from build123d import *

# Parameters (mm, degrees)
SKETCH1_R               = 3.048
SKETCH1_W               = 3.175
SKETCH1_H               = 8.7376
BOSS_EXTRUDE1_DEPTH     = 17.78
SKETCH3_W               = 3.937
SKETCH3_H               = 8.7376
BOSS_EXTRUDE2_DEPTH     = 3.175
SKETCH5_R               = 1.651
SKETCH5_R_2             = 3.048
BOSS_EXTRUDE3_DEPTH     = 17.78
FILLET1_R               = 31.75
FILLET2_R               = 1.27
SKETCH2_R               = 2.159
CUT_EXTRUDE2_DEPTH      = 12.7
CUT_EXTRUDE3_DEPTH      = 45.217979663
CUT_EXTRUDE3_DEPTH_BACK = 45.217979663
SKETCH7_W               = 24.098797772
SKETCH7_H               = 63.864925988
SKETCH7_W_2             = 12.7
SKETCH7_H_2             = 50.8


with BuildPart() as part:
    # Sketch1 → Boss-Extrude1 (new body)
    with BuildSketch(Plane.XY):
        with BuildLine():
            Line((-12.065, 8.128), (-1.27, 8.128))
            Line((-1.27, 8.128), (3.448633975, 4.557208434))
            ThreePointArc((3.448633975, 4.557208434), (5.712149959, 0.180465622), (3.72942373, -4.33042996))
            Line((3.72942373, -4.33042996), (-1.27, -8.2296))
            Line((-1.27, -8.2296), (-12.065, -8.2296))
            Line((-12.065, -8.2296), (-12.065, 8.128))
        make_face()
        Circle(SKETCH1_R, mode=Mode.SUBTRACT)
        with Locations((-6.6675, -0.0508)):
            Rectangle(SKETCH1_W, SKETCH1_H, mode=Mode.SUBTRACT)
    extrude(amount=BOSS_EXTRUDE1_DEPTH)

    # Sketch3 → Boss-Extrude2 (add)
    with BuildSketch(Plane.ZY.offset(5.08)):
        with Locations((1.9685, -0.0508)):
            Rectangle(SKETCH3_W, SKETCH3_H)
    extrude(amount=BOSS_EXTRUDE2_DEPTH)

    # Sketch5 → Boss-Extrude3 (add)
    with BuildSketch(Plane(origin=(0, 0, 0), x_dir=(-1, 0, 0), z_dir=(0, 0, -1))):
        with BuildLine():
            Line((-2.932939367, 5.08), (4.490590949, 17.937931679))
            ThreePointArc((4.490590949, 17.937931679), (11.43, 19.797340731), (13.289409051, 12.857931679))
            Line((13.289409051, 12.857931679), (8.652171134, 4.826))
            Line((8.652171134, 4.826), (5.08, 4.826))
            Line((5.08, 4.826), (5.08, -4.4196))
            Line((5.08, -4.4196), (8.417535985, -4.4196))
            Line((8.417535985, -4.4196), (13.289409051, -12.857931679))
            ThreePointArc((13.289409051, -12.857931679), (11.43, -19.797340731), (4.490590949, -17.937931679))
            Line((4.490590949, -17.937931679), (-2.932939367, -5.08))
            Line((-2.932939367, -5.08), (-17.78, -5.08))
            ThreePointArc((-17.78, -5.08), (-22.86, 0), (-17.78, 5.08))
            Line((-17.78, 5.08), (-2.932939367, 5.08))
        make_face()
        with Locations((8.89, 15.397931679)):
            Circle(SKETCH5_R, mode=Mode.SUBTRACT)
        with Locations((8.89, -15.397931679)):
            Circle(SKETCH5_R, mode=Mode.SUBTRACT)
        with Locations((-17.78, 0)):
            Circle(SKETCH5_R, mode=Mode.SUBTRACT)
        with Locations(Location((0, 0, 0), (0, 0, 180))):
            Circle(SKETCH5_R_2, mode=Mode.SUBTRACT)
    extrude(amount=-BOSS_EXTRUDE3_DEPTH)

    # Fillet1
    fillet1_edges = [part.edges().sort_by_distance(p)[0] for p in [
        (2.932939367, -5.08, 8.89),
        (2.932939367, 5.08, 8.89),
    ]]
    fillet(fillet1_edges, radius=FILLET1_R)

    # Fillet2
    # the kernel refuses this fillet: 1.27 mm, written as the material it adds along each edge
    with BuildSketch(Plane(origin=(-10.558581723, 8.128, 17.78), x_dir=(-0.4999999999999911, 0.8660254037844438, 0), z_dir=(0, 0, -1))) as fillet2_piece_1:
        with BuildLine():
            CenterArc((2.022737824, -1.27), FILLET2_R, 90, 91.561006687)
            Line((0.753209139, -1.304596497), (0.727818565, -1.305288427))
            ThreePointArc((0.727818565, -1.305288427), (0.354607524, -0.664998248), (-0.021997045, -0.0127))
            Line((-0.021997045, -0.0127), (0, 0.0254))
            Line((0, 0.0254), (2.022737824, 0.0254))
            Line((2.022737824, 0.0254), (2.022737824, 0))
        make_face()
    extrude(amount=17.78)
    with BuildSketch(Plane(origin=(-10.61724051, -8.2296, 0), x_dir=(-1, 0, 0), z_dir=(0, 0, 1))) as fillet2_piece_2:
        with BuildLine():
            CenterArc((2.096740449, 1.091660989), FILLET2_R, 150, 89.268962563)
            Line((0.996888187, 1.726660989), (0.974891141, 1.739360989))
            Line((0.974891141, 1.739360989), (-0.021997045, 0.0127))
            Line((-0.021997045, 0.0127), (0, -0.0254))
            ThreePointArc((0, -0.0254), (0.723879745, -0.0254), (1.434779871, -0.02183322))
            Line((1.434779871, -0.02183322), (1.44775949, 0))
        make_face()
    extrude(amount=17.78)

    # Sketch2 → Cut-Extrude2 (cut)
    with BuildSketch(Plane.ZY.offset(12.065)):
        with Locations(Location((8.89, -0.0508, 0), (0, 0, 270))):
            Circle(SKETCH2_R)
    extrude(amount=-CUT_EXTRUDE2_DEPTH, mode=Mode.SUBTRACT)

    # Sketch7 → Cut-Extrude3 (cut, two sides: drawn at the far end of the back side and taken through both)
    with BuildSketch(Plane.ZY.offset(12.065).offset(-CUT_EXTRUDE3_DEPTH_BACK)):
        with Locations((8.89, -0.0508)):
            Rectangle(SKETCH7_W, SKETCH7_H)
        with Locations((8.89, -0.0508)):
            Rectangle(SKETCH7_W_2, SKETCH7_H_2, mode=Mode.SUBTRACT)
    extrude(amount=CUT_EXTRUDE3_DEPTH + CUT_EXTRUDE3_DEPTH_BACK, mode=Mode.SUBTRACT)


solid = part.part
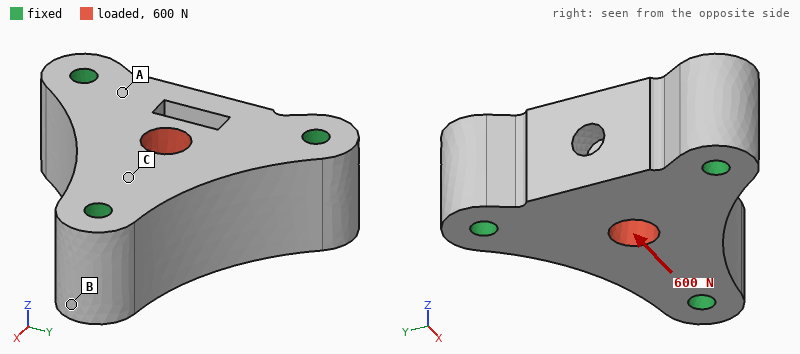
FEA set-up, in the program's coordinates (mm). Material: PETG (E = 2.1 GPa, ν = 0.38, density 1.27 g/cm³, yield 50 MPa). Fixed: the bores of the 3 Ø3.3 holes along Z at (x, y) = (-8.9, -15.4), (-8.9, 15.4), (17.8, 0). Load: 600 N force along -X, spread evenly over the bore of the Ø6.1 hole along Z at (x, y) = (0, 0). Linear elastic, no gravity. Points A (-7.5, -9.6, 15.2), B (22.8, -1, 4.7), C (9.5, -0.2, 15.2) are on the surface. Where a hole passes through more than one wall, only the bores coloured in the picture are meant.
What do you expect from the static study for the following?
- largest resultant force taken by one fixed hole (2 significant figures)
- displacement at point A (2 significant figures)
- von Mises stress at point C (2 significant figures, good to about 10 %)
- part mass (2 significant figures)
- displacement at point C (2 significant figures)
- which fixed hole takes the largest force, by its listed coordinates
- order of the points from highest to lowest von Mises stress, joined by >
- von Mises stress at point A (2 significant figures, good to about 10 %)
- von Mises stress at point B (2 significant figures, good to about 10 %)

330 N
10 µm
2.7 MPa
11 g
9.4 µm
(17.8, 0)
C > A > B
1.7 MPa
0.82 MPa
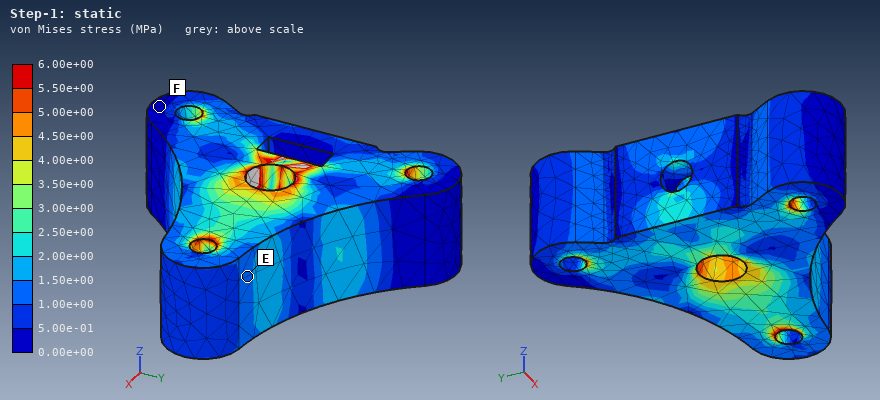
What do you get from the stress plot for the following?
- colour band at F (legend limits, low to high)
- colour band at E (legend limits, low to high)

0.00e+00 to 5.00e-01 MPa
1.00e+00 to 1.50e+00 MPa
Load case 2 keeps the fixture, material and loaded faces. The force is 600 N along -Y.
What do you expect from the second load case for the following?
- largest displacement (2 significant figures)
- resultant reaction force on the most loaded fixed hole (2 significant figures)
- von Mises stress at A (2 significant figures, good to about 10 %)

39 µm
280 N
1.8 MPa
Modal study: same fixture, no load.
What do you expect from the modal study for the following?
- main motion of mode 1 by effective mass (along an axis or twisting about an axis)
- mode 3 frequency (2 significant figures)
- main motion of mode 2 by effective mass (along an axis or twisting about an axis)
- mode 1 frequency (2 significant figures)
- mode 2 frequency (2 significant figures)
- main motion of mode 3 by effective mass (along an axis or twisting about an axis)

along Z
11 kHz
along Y
9100 Hz
9900 Hz
along X
